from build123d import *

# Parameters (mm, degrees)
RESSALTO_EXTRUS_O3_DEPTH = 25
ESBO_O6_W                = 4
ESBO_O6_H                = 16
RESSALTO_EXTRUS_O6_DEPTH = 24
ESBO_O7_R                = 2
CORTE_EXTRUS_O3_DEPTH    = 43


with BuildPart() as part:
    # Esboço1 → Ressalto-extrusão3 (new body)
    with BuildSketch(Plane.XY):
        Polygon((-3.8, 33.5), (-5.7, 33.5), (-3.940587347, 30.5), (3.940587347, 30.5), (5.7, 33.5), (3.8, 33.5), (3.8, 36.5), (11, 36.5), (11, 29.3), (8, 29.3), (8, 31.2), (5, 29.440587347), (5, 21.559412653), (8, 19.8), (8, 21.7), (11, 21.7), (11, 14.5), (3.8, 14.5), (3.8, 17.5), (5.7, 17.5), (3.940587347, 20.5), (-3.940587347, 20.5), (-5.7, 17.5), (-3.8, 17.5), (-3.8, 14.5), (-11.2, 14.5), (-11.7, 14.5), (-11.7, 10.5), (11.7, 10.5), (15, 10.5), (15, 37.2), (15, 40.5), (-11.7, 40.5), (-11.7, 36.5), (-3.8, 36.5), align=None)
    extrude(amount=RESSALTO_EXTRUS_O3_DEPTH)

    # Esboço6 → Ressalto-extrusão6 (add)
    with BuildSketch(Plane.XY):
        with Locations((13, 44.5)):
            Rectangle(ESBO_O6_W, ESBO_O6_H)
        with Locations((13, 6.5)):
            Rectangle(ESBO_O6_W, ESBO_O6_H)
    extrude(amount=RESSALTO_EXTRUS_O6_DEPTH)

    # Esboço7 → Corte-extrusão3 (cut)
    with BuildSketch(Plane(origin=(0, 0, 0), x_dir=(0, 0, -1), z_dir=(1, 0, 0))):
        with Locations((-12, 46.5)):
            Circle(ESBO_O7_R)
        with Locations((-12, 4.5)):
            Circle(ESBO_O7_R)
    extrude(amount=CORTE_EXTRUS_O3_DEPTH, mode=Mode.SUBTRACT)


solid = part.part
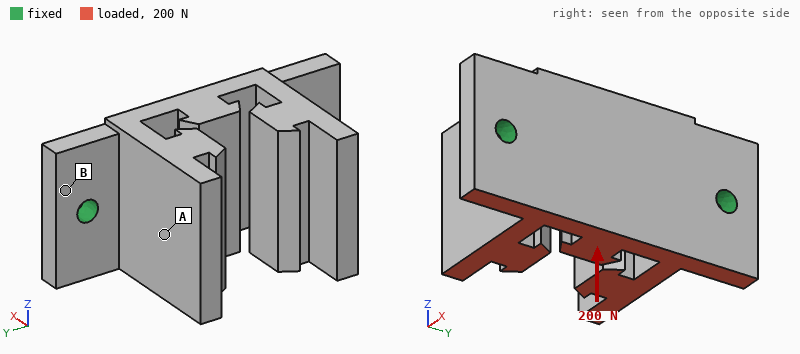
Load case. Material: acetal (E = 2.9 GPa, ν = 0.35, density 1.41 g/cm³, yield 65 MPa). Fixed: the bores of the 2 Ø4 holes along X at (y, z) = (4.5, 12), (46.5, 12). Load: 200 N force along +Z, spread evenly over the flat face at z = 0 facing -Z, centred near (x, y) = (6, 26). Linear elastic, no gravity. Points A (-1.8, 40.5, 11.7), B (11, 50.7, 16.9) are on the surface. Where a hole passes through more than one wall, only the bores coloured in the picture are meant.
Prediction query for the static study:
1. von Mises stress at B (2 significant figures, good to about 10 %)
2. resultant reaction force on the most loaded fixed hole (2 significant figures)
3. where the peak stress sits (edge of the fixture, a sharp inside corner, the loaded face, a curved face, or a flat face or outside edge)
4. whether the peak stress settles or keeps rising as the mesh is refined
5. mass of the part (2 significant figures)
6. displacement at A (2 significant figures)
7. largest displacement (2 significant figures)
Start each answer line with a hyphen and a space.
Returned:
- 4.3 MPa
- 100 N
- edge of the fixture
- keeps rising
- 19 g
- 0.15 mm
- 0.27 mm
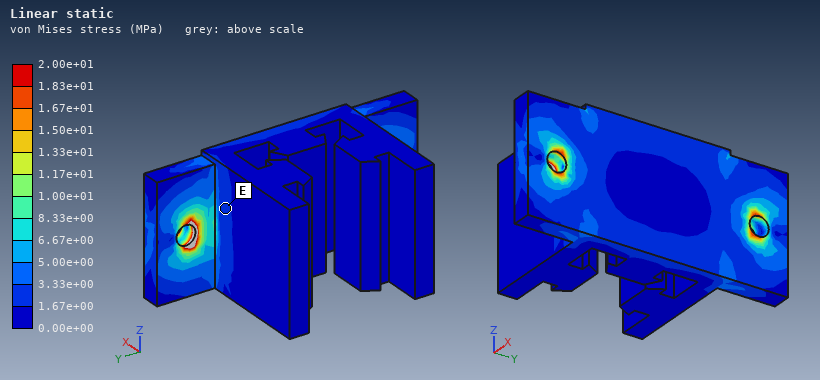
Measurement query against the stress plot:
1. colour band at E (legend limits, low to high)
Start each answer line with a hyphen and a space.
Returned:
- 1.67e+00 to 3.33e+00 MPa
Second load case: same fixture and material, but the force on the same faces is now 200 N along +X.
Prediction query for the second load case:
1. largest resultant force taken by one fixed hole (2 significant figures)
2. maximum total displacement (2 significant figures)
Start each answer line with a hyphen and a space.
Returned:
- 100 N
- 0.51 mm
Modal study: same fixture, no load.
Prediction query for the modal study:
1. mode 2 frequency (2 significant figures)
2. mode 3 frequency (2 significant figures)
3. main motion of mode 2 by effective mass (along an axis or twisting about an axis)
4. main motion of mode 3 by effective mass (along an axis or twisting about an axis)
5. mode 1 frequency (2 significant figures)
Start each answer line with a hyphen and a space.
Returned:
- 1100 Hz
- 1200 Hz
- along Z
- along Y
- 950 Hz
